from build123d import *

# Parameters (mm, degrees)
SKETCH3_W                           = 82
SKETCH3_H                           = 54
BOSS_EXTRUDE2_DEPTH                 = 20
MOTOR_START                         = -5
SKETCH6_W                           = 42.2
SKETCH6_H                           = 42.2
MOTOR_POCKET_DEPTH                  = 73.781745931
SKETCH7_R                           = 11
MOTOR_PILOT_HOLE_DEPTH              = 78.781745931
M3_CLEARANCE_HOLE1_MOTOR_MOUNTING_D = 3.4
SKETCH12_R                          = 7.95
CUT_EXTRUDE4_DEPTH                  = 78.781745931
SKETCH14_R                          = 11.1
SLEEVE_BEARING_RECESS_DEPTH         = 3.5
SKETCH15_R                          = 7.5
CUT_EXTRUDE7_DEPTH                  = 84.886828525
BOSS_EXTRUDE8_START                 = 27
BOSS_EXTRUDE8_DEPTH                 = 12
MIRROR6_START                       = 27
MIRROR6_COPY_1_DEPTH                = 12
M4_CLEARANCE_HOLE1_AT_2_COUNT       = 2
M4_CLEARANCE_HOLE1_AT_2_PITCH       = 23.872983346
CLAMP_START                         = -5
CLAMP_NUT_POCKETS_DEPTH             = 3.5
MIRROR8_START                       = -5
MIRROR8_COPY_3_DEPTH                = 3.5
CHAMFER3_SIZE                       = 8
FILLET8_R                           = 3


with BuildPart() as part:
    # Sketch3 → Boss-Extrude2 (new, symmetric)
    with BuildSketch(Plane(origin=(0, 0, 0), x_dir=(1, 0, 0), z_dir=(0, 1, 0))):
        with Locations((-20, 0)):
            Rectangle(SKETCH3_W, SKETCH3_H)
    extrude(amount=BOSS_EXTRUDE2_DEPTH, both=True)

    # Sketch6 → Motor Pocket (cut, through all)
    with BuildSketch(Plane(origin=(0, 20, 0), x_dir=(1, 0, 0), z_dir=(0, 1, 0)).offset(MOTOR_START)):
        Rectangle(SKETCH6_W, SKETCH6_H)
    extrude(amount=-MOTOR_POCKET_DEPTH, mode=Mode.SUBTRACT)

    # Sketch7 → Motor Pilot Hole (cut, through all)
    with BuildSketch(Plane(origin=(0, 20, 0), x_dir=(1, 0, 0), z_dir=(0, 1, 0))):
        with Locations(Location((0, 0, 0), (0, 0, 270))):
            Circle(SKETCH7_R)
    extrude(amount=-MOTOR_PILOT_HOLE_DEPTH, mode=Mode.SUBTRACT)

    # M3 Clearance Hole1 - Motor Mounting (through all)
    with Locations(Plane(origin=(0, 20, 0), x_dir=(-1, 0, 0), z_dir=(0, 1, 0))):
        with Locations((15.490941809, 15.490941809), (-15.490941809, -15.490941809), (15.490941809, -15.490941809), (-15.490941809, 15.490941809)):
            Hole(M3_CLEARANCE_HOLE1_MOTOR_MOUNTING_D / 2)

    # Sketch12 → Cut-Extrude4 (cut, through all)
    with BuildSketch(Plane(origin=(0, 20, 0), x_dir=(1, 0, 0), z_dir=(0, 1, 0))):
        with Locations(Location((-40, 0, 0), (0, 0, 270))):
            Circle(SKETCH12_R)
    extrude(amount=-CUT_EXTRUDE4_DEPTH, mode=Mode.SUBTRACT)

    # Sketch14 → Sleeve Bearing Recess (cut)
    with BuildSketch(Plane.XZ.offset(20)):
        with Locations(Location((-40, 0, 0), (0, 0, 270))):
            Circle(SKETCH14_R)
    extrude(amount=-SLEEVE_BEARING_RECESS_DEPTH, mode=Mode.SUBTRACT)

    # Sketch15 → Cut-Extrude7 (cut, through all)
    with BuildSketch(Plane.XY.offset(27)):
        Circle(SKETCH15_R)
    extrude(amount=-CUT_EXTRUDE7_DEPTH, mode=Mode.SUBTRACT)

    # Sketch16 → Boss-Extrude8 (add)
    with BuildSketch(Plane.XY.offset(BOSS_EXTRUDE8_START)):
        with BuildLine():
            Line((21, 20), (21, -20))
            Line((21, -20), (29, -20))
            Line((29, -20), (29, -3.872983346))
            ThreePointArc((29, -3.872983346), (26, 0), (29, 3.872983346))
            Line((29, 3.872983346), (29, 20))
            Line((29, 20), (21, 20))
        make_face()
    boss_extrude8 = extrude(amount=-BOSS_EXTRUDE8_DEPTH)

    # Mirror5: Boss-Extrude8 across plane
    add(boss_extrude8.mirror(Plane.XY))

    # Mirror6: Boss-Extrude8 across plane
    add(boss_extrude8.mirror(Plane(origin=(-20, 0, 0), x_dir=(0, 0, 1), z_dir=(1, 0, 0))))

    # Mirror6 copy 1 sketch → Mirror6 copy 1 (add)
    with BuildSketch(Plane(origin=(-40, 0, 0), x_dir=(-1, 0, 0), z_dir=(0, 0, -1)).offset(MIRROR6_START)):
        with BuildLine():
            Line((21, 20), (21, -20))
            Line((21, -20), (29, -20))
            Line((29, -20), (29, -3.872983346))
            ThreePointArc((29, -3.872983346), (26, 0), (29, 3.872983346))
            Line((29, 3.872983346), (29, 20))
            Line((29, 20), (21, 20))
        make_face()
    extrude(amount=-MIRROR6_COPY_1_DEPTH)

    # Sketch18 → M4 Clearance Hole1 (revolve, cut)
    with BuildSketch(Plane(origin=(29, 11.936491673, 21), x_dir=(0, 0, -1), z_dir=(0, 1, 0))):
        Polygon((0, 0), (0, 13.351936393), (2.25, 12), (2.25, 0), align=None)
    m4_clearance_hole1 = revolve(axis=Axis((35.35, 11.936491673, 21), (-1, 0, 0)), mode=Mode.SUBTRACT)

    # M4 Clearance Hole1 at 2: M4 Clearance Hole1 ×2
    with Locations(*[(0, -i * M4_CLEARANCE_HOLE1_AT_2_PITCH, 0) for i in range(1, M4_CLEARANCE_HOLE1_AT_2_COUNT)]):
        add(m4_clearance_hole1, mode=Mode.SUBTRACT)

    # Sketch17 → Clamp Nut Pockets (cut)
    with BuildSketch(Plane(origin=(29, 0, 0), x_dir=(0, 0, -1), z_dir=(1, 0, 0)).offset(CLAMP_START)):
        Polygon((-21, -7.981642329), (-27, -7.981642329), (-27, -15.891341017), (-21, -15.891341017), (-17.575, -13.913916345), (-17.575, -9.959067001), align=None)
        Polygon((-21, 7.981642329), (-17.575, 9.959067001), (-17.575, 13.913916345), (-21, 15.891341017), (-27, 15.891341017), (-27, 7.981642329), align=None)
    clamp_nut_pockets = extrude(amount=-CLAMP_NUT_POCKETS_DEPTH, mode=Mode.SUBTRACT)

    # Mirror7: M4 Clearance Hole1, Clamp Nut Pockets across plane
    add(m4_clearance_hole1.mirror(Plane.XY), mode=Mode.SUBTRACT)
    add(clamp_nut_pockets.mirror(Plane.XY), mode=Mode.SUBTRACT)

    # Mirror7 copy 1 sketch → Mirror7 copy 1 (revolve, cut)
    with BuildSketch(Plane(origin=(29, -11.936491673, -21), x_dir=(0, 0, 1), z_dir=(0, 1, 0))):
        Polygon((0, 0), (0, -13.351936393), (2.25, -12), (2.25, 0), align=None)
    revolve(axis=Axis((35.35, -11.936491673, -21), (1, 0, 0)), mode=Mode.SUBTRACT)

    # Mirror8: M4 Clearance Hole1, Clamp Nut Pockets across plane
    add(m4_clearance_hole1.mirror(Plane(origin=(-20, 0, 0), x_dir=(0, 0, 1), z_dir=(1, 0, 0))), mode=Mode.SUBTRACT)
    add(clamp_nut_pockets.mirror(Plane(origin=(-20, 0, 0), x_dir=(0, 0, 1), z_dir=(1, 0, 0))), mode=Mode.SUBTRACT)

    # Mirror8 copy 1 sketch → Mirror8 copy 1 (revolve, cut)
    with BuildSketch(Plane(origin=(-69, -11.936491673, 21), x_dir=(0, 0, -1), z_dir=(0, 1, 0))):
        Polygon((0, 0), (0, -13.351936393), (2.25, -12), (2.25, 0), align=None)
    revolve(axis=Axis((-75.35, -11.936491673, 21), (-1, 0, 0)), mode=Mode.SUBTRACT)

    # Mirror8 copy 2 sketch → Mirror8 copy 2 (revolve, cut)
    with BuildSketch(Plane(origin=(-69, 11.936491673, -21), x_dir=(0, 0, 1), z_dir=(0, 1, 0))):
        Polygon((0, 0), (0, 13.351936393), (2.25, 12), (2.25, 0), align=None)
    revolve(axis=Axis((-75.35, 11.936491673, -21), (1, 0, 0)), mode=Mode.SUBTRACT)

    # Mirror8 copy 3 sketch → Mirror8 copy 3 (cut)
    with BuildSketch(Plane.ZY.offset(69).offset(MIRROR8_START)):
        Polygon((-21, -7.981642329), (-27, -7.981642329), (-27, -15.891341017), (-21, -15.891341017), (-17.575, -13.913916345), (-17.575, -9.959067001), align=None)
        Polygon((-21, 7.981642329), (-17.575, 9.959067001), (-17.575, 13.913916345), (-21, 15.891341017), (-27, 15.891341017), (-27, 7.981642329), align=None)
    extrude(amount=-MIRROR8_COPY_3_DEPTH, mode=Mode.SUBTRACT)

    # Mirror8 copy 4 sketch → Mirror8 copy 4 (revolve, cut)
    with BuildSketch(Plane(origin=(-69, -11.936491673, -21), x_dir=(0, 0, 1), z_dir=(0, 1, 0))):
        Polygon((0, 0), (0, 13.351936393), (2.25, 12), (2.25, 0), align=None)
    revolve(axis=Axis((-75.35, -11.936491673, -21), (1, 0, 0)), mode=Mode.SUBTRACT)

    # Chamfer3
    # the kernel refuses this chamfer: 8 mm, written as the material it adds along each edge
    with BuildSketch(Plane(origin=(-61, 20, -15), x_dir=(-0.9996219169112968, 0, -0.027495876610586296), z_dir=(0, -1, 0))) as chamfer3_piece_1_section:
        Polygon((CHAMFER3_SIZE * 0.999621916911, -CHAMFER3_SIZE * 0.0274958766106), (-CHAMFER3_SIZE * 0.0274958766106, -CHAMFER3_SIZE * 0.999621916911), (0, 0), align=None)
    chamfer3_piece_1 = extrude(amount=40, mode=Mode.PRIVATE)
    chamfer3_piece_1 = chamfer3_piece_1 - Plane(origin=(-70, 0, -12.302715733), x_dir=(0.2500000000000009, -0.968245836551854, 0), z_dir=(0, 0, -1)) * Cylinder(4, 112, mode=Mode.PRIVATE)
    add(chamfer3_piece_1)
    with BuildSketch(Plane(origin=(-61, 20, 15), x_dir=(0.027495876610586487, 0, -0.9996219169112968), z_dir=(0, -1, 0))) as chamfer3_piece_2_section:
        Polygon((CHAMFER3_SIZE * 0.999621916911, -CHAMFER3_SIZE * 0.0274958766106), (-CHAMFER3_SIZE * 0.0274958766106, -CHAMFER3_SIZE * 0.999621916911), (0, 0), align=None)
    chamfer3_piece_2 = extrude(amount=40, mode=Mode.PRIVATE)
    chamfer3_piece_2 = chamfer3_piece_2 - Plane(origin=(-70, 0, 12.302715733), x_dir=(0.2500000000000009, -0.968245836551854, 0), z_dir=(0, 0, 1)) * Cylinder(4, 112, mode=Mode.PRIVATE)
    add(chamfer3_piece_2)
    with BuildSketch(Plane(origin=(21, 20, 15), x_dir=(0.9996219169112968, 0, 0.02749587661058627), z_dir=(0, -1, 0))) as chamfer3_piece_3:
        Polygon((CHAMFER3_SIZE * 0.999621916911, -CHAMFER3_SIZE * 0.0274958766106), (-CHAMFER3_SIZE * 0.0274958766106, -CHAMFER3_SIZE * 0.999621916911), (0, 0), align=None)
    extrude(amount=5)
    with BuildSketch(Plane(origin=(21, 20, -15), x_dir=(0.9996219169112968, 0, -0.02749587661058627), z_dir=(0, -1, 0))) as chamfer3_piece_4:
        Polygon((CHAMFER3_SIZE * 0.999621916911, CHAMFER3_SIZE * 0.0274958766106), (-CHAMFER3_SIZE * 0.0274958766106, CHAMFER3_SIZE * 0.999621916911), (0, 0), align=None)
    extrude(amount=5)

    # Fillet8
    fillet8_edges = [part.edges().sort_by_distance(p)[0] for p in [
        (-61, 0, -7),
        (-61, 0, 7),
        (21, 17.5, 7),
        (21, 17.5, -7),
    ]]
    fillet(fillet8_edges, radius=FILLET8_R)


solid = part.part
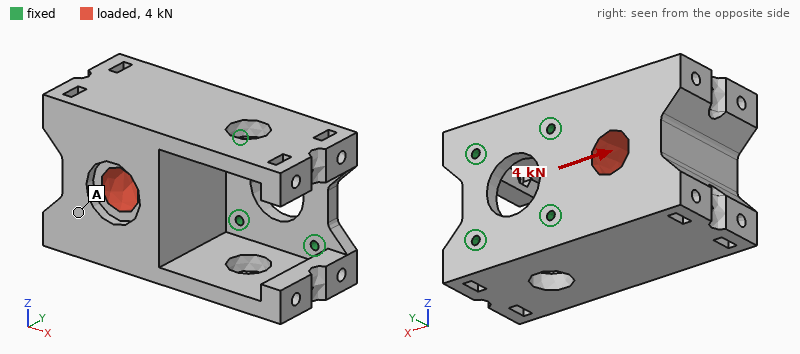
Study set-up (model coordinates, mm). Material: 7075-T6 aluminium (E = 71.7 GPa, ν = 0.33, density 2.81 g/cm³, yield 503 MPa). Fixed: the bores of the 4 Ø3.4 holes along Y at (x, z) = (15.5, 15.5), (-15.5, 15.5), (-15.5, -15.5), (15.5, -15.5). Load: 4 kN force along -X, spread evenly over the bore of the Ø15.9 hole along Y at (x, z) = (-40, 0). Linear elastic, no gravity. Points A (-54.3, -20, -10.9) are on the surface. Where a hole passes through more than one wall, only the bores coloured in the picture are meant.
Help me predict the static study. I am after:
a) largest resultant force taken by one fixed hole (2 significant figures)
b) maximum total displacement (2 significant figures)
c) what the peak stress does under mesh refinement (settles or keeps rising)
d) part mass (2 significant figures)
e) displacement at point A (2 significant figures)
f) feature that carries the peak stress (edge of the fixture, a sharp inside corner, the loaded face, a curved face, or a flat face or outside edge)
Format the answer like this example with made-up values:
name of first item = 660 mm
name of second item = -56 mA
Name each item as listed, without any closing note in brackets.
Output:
largest resultant force taken by one fixed hole = 1.6 kN
maximum total displacement = 61 µm
what the peak stress does under mesh refinement = keeps rising
part mass = 330 g
displacement at point A = 51 µm
feature that carries the peak stress = edge of the fixture
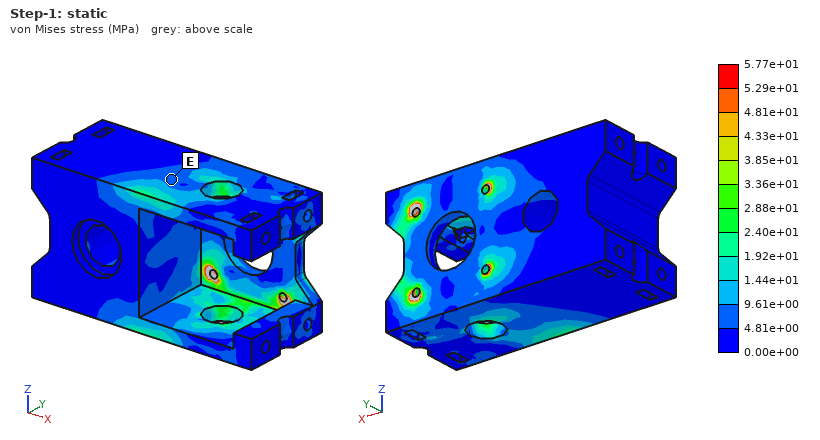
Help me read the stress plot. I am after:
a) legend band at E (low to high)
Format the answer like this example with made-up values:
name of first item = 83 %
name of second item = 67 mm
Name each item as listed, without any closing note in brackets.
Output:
legend band at E = 4.81e+00 to 9.61e+00 MPa
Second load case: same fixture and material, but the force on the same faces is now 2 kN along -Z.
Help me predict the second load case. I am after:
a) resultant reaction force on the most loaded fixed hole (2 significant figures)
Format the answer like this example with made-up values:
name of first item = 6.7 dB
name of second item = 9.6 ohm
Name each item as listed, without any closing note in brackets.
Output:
resultant reaction force on the most loaded fixed hole = 1.6 kN
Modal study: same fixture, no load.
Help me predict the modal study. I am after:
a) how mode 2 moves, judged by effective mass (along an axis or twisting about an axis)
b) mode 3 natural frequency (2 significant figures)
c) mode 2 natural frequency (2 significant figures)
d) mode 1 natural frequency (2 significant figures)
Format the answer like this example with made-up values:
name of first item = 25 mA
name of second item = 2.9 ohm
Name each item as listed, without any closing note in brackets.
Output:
how mode 2 moves, judged by effective mass = along Z
mode 3 natural frequency = 4000 Hz
mode 2 natural frequency = 3000 Hz
mode 1 natural frequency = 2000 Hz
